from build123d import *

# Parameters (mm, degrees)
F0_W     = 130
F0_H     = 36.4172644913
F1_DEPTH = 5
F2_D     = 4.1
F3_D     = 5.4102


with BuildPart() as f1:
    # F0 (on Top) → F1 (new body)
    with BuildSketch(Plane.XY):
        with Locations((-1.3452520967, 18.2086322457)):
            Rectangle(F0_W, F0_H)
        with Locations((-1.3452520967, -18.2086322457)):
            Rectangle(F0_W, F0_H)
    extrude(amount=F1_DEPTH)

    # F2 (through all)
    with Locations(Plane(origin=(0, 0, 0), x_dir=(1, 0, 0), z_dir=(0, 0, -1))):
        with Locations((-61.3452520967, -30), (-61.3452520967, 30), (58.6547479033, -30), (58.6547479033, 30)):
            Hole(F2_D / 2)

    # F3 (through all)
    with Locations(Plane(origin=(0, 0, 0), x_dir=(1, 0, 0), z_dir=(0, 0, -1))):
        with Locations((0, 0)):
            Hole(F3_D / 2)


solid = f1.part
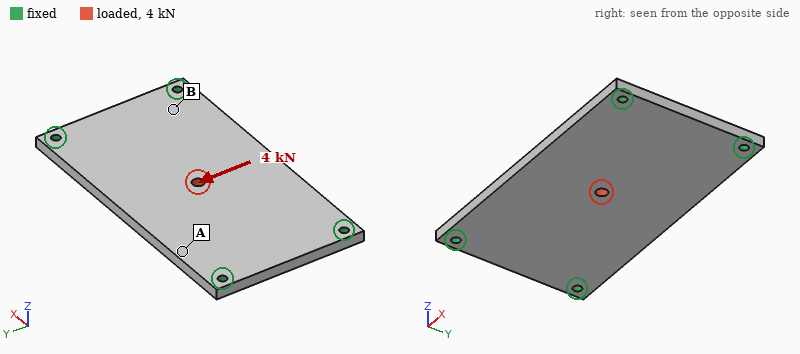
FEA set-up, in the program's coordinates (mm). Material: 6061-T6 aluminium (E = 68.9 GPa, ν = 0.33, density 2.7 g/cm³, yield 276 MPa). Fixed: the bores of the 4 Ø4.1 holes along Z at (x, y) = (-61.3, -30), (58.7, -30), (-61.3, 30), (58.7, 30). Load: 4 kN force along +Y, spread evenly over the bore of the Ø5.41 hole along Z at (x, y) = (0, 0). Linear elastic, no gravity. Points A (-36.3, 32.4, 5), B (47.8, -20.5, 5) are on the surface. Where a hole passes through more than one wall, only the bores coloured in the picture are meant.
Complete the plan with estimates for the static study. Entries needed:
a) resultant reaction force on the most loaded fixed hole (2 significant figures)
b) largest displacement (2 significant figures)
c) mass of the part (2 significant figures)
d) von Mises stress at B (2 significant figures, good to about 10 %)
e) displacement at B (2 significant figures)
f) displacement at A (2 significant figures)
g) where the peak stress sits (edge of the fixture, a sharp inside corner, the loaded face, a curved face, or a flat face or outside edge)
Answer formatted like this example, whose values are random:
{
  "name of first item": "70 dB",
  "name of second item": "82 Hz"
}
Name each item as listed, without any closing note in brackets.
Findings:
{
  "resultant reaction force on the most loaded fixed hole": "1.4 kN",
  "largest displacement": "24 µm",
  "mass of the part": "130 g",
  "von Mises stress at B": "14 MPa",
  "displacement at B": "4.6 µm",
  "displacement at A": "9.8 µm",
  "where the peak stress sits": "the loaded face"
}
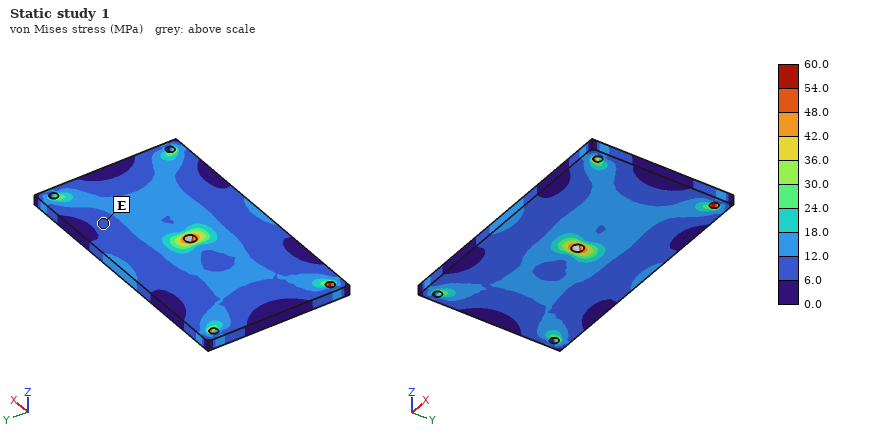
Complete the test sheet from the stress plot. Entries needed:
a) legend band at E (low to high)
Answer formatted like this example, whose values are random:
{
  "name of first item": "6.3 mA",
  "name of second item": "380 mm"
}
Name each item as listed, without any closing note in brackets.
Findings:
{
  "legend band at E": "6.0 to 12.0 MPa"
}
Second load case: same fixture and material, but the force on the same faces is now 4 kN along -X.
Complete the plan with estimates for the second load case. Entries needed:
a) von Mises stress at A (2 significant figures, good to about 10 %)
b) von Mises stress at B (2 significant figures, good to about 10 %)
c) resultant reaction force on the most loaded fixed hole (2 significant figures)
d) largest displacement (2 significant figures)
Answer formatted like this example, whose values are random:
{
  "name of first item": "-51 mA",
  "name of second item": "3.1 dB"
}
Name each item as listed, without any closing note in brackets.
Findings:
{
  "von Mises stress at A": "6.4 MPa",
  "von Mises stress at B": "9.5 MPa",
  "resultant reaction force on the most loaded fixed hole": "1.1 kN",
  "largest displacement": "13 µm"
}
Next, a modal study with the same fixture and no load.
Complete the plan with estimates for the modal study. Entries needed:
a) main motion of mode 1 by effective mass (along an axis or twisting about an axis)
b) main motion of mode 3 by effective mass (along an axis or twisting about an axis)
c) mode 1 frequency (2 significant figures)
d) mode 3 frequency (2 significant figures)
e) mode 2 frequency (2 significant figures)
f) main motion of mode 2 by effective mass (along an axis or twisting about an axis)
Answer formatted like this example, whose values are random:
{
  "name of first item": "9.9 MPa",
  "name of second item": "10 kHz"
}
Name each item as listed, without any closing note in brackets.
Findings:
{
  "main motion of mode 1 by effective mass": "along Z",
  "main motion of mode 3 by effective mass": "twisting about Y",
  "mode 1 frequency": "1500 Hz",
  "mode 3 frequency": "4100 Hz",
  "mode 2 frequency": "2600 Hz",
  "main motion of mode 2 by effective mass": "twisting about X"
}
